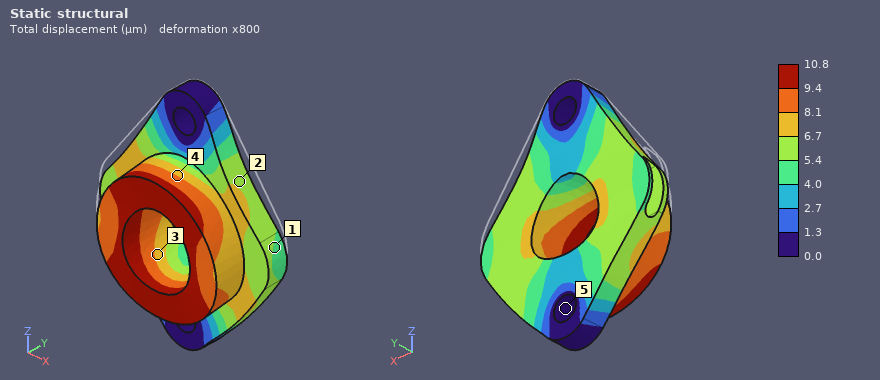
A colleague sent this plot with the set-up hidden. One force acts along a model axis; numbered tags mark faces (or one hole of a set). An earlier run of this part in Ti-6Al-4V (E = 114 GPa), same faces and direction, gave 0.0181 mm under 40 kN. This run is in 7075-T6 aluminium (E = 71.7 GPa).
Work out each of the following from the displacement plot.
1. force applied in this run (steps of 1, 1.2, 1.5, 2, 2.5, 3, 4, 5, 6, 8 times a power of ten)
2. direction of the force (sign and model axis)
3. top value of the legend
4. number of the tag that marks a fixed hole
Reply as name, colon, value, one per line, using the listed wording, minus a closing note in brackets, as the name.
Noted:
force applied in this run: 15 kN
direction of the force: -Z
top value of the legend: 10.8 µm
number of the tag that marks a fixed hole: 5
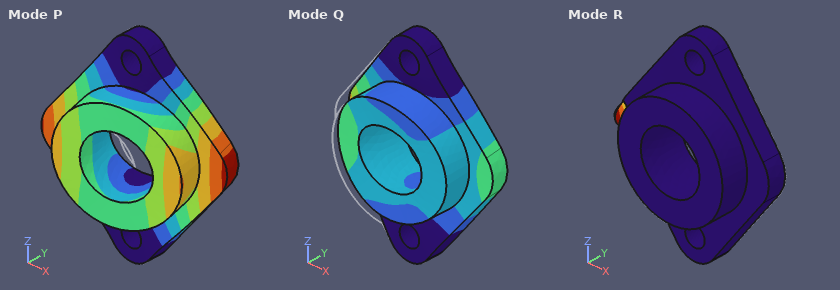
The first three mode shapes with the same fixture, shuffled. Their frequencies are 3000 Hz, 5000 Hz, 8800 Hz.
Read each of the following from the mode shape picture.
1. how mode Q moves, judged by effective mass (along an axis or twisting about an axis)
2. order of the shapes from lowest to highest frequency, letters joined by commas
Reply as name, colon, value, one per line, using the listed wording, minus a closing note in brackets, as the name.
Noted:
how mode Q moves, judged by effective mass: along Y
order of the shapes from lowest to highest frequency, letters joined by commas: P, Q, R
